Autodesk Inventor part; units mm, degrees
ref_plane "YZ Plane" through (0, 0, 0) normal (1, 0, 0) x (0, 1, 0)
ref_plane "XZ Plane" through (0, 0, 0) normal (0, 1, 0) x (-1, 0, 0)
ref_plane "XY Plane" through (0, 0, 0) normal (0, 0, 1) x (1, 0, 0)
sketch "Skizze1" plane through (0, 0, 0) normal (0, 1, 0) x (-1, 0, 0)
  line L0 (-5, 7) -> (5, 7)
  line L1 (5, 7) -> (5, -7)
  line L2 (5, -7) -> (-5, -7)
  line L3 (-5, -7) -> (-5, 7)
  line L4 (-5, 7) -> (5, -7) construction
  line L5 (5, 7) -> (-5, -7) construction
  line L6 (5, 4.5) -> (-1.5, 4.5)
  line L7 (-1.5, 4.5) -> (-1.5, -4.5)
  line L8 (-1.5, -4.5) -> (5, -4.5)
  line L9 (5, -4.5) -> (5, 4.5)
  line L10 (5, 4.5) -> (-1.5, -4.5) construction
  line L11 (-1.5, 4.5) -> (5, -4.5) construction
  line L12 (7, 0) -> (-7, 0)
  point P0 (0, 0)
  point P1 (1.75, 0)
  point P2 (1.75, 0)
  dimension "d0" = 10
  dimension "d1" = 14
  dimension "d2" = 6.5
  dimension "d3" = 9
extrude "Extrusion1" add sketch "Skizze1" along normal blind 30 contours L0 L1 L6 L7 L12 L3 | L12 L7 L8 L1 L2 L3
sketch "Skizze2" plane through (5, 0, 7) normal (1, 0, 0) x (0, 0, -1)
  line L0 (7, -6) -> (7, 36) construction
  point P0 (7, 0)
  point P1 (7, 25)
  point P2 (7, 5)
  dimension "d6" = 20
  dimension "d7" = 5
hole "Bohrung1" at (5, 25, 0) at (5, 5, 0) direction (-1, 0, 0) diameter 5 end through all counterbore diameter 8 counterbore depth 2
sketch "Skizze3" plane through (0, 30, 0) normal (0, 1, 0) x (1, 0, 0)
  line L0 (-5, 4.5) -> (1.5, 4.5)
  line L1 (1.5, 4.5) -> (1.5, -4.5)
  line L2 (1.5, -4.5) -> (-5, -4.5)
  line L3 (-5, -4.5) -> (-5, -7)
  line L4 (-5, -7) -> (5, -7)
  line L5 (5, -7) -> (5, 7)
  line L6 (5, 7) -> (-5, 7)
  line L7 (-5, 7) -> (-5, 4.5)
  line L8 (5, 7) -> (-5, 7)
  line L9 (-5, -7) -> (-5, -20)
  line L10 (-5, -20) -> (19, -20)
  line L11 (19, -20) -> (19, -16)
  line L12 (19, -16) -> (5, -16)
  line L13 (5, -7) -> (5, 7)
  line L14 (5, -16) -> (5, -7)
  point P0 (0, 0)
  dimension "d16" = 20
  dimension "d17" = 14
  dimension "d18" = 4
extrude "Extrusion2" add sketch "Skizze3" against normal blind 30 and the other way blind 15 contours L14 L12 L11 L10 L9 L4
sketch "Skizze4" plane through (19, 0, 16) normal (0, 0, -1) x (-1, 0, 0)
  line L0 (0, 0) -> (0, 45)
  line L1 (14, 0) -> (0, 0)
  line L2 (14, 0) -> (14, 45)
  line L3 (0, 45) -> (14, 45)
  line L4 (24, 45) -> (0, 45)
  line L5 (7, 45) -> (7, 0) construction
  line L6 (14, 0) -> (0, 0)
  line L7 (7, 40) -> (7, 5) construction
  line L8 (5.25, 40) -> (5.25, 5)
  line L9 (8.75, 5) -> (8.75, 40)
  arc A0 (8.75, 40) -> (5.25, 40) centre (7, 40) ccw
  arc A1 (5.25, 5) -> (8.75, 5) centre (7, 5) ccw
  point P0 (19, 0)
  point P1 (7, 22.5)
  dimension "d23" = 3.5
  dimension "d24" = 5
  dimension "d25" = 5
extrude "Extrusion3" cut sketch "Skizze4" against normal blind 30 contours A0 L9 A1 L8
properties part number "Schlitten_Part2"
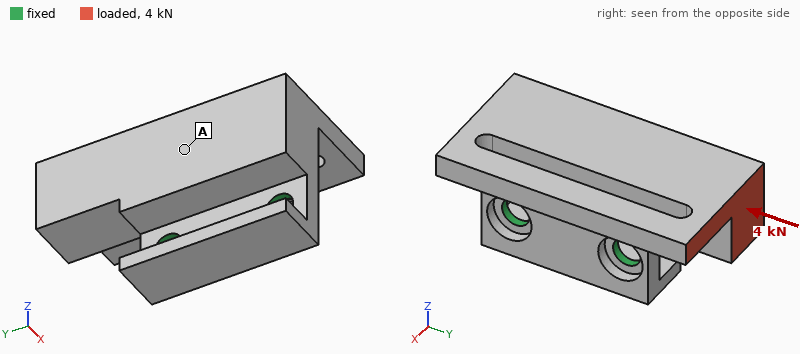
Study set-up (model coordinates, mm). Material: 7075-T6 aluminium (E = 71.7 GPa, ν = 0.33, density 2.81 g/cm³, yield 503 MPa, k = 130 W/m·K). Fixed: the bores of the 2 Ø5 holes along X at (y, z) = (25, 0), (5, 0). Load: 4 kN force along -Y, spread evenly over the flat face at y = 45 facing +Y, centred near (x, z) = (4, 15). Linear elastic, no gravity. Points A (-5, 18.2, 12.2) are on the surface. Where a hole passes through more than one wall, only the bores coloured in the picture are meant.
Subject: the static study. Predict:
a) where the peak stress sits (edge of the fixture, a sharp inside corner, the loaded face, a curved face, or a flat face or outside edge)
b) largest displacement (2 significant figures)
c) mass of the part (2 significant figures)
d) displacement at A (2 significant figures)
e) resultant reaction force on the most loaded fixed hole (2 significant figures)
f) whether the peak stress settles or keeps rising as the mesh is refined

edge of the fixture
0.11 mm
28 g
0.019 mm
3.3 kN
keeps rising
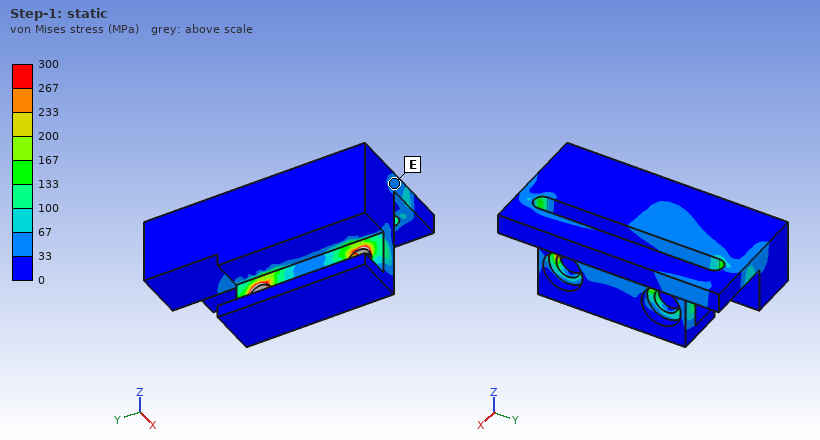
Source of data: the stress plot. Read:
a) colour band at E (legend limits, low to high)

33 to 67 MPa
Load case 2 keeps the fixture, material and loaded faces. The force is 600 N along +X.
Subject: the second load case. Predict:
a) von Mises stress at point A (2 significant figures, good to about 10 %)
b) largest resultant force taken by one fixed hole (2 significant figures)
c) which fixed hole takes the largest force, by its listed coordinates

45 MPa
1.2 kN
(25, 0)
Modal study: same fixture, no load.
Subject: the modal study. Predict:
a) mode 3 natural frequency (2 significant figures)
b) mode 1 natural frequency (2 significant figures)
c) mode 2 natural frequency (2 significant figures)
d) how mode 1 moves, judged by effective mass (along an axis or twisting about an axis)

6300 Hz
2000 Hz
5200 Hz
along X
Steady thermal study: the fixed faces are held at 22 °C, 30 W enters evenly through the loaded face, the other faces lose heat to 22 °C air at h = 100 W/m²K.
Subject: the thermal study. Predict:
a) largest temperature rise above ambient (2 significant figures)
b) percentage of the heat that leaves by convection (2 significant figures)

50 K
31 %
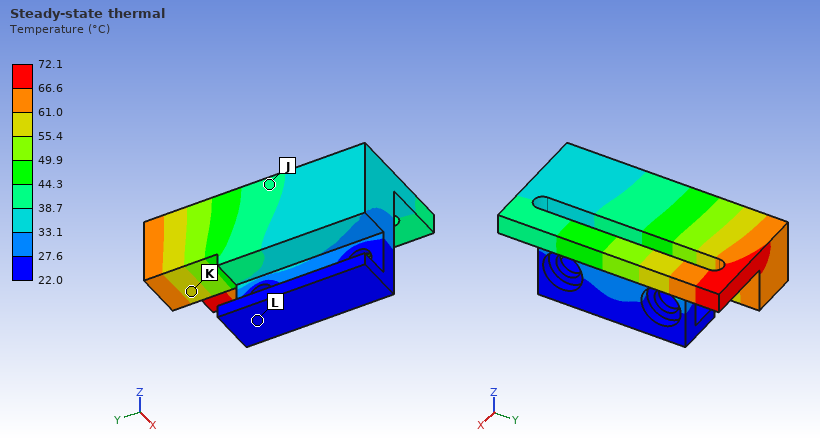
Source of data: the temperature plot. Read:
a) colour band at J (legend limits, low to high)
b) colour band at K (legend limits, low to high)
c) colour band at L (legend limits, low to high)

38.7 to 44.3 °C
55.4 to 61.0 °C
22.0 to 27.6 °C
